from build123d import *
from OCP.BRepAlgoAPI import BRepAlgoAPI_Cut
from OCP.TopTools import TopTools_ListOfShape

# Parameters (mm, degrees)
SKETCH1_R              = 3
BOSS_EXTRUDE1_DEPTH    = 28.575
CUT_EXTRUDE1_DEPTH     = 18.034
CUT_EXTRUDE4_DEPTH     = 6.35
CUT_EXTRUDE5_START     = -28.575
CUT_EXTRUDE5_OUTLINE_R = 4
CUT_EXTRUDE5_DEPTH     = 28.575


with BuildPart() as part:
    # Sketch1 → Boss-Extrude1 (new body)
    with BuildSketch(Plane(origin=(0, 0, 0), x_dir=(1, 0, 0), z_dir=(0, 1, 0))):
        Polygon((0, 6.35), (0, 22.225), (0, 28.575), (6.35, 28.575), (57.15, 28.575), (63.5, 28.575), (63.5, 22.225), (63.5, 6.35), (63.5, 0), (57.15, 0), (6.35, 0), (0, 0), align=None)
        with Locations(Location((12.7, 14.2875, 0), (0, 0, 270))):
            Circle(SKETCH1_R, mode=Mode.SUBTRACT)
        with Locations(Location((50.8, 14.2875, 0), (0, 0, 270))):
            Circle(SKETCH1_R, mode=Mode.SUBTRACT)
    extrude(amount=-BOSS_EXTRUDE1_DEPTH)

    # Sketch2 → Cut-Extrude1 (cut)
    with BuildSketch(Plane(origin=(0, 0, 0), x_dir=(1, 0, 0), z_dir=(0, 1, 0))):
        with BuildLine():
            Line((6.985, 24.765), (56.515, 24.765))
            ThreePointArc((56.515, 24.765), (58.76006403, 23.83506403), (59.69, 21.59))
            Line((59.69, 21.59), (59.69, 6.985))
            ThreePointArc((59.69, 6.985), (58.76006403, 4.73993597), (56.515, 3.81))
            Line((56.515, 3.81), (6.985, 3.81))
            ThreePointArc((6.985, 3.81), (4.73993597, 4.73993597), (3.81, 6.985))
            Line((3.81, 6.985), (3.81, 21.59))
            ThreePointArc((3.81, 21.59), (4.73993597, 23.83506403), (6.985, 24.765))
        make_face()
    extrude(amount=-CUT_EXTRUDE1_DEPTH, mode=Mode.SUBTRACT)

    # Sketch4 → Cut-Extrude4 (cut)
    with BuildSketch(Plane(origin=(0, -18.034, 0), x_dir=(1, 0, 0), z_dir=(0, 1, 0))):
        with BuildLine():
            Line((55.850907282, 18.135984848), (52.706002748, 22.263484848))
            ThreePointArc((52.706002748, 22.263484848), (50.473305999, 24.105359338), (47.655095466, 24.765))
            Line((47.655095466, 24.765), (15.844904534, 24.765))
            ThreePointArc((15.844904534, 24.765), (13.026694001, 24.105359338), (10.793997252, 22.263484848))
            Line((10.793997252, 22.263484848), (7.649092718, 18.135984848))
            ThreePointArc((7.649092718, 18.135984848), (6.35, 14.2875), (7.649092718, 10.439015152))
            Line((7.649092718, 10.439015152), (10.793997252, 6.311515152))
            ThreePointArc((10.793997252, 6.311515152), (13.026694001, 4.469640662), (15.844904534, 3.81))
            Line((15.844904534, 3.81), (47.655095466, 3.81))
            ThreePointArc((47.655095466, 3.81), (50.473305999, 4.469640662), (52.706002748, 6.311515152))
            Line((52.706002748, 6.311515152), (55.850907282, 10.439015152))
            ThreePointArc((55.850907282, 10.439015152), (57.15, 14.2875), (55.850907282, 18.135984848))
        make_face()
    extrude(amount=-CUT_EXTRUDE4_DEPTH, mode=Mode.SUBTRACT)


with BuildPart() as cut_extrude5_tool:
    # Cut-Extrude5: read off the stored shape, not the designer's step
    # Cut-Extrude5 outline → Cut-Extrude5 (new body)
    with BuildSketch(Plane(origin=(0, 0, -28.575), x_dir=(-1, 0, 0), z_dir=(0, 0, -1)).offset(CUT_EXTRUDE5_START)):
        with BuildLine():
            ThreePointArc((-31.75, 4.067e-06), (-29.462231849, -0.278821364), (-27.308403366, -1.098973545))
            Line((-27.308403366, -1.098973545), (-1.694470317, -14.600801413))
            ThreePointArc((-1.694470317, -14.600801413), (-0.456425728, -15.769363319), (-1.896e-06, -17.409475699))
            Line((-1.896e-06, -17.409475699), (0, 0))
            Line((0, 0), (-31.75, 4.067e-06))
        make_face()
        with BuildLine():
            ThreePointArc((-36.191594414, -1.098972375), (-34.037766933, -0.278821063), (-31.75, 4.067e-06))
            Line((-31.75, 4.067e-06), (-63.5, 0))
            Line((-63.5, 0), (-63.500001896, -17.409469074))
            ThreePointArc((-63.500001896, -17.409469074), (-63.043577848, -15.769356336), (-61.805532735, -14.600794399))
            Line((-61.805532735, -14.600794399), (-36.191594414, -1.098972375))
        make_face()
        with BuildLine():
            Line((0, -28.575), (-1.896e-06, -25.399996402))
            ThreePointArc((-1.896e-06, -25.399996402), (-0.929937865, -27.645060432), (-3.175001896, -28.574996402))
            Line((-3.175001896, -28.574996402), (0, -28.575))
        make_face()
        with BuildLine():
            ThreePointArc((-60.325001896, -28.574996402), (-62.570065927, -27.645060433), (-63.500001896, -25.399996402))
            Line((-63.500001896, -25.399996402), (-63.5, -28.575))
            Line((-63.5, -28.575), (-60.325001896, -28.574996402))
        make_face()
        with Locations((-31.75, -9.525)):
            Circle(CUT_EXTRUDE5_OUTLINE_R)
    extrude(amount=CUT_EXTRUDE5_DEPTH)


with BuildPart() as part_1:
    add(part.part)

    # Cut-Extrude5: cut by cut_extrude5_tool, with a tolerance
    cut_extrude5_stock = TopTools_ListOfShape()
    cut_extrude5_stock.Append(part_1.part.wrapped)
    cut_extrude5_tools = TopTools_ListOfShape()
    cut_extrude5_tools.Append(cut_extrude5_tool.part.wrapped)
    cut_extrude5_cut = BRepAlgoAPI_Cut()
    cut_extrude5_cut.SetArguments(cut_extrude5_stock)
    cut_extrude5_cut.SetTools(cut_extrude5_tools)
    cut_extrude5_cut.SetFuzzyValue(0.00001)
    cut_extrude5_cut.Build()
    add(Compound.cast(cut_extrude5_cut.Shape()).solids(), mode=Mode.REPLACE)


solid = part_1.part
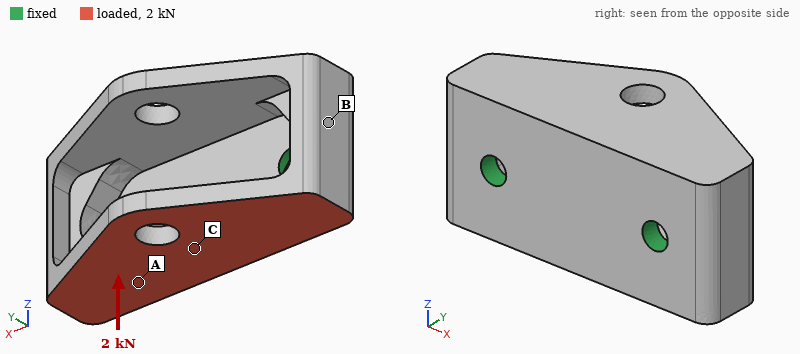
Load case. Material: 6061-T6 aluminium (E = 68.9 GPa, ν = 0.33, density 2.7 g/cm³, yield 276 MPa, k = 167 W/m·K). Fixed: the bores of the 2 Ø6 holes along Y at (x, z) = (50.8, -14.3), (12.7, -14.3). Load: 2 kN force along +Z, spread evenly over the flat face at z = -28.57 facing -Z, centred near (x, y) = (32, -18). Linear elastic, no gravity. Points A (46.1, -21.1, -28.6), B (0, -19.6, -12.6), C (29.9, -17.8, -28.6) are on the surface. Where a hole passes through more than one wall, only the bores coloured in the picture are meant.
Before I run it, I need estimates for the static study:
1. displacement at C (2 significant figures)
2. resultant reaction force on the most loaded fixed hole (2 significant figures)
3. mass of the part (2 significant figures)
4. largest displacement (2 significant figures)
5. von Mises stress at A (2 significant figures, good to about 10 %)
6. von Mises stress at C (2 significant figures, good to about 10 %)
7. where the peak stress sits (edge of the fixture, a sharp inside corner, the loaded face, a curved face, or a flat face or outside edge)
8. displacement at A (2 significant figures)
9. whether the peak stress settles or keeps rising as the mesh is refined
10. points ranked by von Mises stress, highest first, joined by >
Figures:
0.064 mm
1.0 kN
49 g
0.20 mm
52 MPa
28 MPa
edge of the fixture
0.040 mm
keeps rising
A > C > B
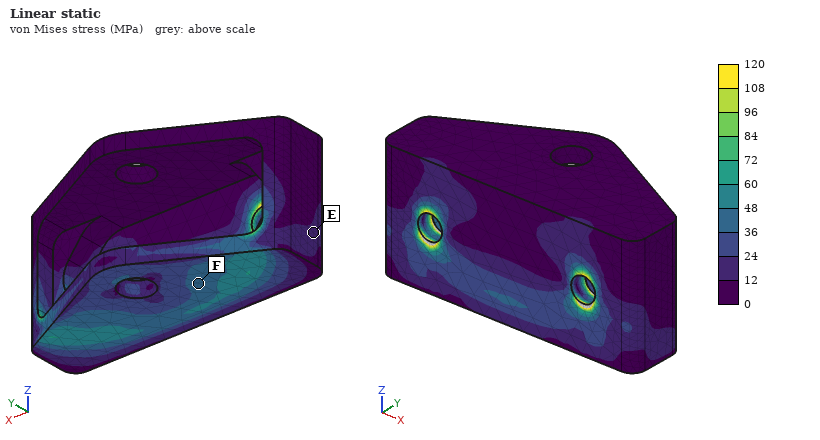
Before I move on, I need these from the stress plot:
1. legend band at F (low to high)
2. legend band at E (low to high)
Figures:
36 to 48 MPa
12 to 24 MPa
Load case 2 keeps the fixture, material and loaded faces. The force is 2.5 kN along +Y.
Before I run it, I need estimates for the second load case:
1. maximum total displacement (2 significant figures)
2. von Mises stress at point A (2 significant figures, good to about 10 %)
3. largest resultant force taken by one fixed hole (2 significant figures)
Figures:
0.17 mm
33 MPa
1.3 kN
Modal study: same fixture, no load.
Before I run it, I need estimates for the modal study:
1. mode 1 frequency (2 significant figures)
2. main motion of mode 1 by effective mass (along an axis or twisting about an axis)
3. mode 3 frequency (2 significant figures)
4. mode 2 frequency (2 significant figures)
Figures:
5000 Hz
along Z
8000 Hz
6800 Hz
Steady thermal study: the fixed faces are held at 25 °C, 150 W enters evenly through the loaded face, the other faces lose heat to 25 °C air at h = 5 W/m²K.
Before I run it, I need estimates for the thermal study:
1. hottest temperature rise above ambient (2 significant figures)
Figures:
80 K
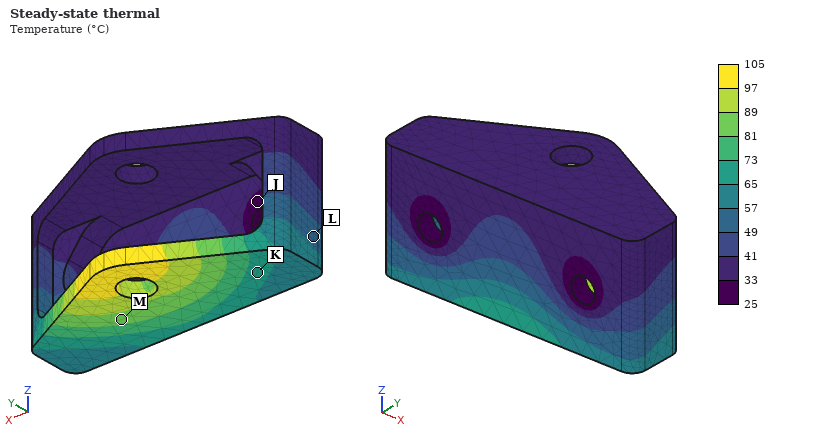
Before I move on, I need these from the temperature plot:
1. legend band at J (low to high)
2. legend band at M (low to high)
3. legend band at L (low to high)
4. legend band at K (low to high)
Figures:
25 to 33 °C
81 to 89 °C
49 to 57 °C
65 to 73 °C
